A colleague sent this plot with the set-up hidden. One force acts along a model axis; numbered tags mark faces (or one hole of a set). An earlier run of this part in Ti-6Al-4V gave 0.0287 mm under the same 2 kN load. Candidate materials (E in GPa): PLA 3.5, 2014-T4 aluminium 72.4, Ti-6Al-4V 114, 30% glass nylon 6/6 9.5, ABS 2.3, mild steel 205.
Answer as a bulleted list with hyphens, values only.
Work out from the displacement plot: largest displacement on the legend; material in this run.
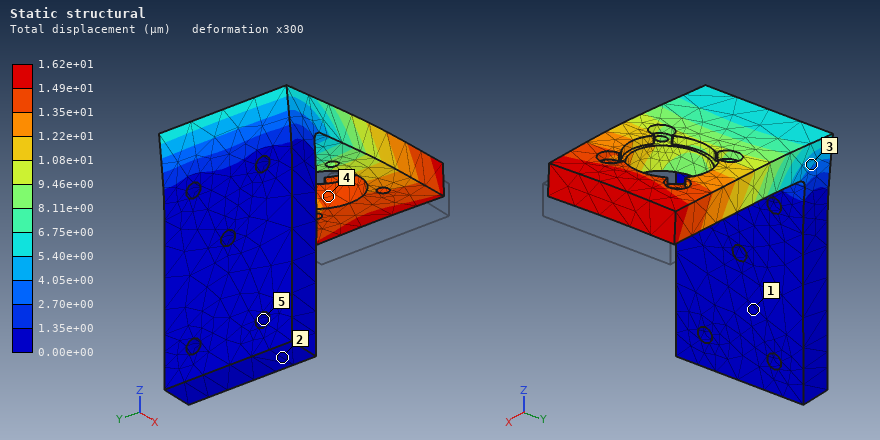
- 1.62e+01 µm
- mild steel
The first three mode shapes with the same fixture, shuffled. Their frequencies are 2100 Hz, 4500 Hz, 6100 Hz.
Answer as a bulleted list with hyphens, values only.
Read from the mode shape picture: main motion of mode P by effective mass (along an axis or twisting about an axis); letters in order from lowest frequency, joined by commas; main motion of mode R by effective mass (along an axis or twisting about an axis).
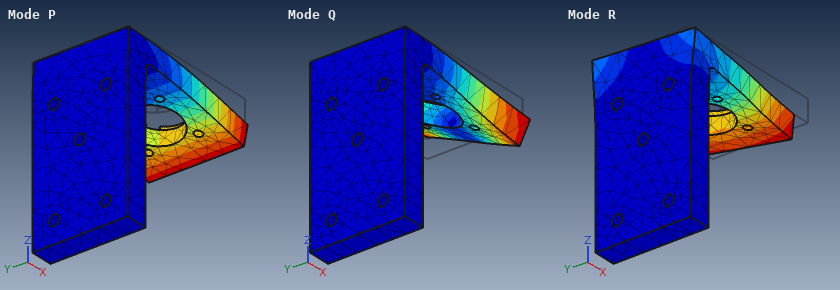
- along Z
- P, R, Q
- along Y
